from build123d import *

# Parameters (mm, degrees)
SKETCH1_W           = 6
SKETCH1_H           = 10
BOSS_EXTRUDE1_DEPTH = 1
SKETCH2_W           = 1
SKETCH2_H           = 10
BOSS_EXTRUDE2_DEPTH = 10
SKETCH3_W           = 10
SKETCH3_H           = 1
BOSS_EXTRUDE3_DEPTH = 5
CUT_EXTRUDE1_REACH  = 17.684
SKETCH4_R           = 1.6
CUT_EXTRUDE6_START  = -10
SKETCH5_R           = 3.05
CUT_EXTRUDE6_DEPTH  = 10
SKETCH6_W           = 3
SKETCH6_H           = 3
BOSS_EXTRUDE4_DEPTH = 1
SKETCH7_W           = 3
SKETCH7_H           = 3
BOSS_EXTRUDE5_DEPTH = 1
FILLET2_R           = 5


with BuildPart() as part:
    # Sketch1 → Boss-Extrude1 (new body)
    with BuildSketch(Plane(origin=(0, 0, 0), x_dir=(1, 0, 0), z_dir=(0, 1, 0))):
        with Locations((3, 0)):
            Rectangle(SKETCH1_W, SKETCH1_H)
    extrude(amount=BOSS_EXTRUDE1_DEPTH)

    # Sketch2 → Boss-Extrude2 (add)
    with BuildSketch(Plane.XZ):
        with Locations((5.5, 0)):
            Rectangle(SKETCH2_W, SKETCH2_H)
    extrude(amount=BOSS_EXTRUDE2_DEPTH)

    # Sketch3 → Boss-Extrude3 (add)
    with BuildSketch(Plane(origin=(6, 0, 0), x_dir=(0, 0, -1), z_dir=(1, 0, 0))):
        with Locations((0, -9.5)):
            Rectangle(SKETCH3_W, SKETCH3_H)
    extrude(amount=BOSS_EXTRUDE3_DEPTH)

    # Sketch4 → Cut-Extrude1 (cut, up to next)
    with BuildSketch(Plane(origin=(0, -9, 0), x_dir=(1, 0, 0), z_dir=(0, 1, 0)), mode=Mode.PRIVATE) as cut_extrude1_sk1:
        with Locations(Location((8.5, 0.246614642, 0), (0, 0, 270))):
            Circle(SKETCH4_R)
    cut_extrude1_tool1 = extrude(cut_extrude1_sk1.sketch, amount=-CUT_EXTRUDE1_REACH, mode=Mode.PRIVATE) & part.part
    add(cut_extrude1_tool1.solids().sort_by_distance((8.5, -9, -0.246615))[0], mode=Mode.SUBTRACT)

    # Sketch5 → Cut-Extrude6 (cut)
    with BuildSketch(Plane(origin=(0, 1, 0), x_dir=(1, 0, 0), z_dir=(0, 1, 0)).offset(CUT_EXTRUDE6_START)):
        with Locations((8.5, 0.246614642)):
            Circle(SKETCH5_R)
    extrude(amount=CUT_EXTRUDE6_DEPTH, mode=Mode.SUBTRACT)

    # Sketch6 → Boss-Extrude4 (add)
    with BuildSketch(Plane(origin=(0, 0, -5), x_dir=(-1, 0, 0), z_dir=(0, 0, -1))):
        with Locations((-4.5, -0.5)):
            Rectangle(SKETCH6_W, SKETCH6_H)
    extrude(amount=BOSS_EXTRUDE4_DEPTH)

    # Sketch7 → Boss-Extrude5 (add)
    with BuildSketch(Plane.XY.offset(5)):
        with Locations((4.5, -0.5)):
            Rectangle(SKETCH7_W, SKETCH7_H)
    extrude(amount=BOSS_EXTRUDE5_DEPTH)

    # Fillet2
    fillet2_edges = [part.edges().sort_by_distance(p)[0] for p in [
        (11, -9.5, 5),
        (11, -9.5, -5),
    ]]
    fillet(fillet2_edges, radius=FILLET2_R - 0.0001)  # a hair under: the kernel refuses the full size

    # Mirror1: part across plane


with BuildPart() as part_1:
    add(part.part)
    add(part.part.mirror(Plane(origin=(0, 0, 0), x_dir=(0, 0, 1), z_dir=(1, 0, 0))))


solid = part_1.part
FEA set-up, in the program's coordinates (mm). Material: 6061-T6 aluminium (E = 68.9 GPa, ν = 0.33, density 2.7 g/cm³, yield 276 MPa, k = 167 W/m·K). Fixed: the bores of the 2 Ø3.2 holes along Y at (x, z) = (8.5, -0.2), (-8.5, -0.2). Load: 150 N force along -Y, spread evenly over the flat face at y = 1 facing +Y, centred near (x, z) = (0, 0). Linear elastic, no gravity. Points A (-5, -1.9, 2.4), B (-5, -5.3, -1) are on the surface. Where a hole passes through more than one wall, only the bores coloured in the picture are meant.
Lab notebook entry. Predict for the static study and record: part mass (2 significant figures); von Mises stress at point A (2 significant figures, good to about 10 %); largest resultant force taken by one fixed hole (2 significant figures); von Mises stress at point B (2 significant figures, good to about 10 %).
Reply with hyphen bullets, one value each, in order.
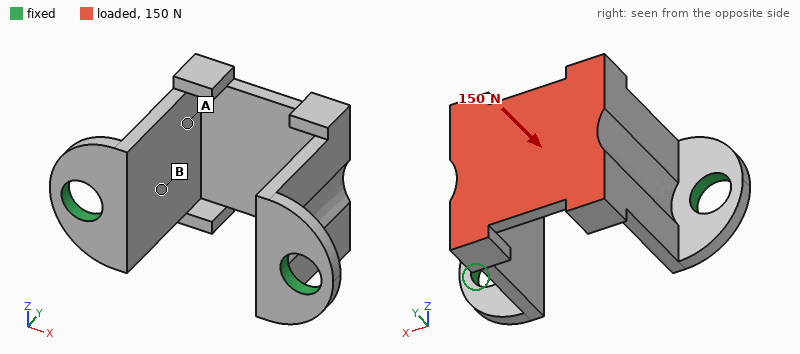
- 1.1 g
- 39 MPa
- 76 N
- 16 MPa
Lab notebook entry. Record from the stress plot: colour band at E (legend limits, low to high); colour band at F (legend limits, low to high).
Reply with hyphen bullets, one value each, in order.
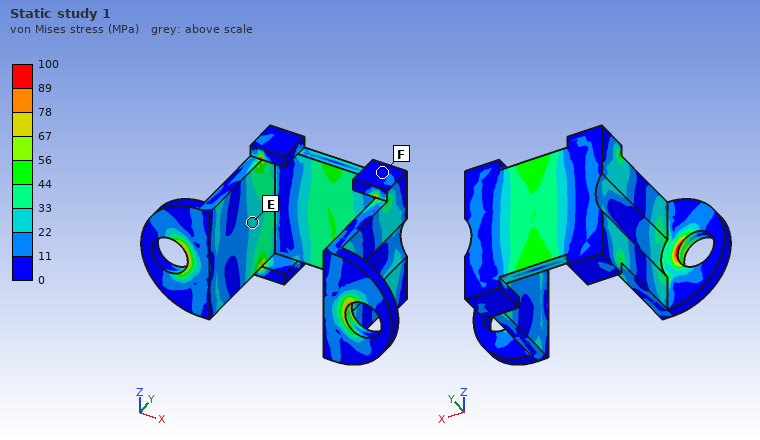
- 22 to 33 MPa
- 0 to 11 MPa
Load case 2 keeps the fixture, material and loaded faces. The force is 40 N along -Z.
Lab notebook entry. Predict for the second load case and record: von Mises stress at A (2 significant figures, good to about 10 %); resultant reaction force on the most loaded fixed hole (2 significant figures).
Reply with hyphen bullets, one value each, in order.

- 9.6 MPa
- 20 N
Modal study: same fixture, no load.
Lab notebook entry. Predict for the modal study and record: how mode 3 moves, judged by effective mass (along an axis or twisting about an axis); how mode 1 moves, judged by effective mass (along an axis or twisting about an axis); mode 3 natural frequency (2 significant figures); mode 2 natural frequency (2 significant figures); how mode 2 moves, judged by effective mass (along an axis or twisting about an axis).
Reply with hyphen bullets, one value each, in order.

- twisting about Y
- along X
- 9400 Hz
- 7300 Hz
- along Z
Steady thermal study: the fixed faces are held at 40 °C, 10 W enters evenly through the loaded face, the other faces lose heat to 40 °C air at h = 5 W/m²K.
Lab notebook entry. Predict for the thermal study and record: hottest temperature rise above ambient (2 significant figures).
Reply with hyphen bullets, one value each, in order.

- 45 K
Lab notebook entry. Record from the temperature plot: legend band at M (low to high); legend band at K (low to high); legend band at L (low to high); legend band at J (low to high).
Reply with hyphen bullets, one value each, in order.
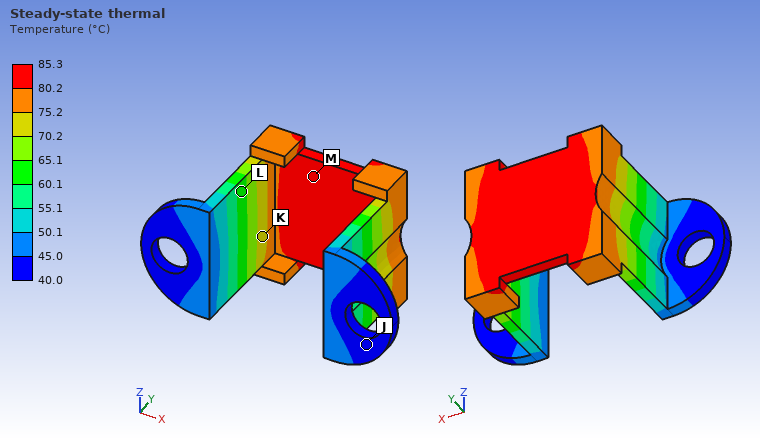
- 80.2 to 85.3 °C
- 70.2 to 75.2 °C
- 60.1 to 65.1 °C
- 40.0 to 45.0 °C
